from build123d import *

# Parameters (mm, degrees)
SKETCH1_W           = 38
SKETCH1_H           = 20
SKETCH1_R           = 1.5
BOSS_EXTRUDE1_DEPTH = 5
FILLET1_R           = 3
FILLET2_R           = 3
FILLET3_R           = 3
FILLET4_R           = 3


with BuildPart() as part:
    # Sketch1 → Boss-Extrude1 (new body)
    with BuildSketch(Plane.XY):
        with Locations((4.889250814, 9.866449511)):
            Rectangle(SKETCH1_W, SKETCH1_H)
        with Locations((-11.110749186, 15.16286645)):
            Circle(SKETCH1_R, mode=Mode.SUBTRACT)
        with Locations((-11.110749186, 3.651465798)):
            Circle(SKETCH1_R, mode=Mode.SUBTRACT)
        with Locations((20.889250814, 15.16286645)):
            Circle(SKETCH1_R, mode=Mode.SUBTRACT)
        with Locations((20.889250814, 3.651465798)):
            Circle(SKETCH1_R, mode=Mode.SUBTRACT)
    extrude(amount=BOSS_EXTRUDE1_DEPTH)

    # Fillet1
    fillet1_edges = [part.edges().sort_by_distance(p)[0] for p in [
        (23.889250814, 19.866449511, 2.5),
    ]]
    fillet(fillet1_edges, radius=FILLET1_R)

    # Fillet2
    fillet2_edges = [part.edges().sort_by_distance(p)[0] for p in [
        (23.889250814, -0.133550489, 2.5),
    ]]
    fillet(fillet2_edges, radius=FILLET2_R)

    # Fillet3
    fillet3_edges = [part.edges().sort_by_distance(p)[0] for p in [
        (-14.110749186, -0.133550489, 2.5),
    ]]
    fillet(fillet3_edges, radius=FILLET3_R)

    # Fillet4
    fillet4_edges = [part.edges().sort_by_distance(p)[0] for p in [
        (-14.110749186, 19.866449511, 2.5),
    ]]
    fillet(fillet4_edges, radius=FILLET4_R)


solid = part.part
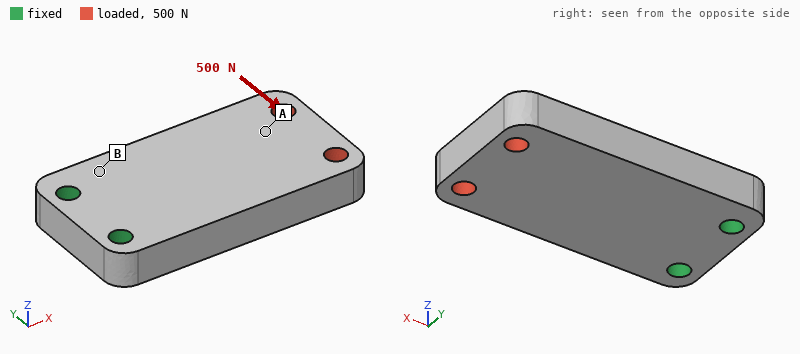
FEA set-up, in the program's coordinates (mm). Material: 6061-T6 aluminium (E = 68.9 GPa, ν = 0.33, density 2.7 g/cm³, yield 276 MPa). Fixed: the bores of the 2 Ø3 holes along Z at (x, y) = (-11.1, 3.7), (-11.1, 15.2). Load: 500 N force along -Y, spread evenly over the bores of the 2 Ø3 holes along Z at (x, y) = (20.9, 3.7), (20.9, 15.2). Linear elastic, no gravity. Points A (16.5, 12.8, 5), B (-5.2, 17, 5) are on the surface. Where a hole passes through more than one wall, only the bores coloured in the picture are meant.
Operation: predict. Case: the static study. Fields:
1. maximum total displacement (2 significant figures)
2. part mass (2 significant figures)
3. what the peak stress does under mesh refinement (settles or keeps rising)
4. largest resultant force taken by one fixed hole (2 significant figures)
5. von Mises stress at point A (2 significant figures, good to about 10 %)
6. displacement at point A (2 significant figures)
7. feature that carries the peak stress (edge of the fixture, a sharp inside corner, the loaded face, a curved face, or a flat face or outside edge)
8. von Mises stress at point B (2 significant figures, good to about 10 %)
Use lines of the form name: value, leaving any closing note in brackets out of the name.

maximum total displacement: 38 µm
part mass: 9.8 g
what the peak stress does under mesh refinement: keeps rising
largest resultant force taken by one fixed hole: 1.2 kN
von Mises stress at point A: 12 MPa
displacement at point A: 27 µm
feature that carries the peak stress: edge of the fixture
von Mises stress at point B: 29 MPa
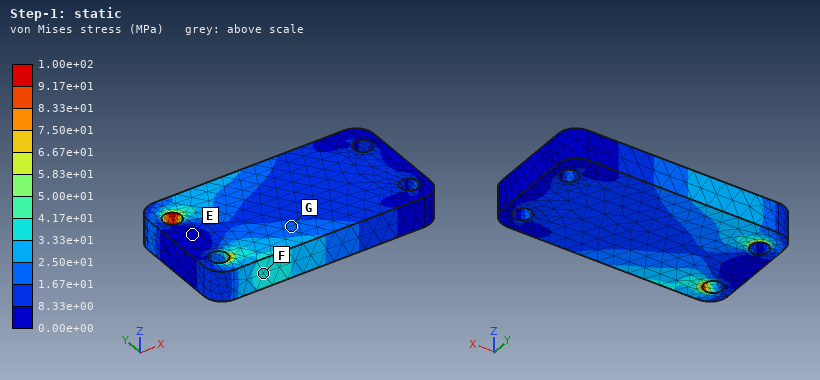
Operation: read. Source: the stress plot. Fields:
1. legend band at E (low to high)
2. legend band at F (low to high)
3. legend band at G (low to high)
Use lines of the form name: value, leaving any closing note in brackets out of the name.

legend band at E: 0.00e+00 to 8.33e+00 MPa
legend band at F: 3.33e+01 to 4.17e+01 MPa
legend band at G: 1.67e+01 to 2.50e+01 MPa
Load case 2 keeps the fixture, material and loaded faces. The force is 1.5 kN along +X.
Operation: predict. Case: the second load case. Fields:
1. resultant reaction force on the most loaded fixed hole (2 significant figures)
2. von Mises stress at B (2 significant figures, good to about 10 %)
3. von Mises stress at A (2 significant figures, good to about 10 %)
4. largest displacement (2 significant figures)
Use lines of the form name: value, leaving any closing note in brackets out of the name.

resultant reaction force on the most loaded fixed hole: 760 N
von Mises stress at B: 15 MPa
von Mises stress at A: 15 MPa
largest displacement: 9.9 µm
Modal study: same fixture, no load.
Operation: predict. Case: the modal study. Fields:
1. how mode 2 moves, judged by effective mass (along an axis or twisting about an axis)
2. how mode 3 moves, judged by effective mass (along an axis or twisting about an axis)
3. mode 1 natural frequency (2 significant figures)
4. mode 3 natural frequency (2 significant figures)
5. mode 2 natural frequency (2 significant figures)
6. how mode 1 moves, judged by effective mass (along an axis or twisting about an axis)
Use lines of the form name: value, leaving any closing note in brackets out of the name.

how mode 2 moves, judged by effective mass: along Y
how mode 3 moves, judged by effective mass: twisting about X
mode 1 natural frequency: 3500 Hz
mode 3 natural frequency: 12 kHz
mode 2 natural frequency: 11 kHz
how mode 1 moves, judged by effective mass: along Z
